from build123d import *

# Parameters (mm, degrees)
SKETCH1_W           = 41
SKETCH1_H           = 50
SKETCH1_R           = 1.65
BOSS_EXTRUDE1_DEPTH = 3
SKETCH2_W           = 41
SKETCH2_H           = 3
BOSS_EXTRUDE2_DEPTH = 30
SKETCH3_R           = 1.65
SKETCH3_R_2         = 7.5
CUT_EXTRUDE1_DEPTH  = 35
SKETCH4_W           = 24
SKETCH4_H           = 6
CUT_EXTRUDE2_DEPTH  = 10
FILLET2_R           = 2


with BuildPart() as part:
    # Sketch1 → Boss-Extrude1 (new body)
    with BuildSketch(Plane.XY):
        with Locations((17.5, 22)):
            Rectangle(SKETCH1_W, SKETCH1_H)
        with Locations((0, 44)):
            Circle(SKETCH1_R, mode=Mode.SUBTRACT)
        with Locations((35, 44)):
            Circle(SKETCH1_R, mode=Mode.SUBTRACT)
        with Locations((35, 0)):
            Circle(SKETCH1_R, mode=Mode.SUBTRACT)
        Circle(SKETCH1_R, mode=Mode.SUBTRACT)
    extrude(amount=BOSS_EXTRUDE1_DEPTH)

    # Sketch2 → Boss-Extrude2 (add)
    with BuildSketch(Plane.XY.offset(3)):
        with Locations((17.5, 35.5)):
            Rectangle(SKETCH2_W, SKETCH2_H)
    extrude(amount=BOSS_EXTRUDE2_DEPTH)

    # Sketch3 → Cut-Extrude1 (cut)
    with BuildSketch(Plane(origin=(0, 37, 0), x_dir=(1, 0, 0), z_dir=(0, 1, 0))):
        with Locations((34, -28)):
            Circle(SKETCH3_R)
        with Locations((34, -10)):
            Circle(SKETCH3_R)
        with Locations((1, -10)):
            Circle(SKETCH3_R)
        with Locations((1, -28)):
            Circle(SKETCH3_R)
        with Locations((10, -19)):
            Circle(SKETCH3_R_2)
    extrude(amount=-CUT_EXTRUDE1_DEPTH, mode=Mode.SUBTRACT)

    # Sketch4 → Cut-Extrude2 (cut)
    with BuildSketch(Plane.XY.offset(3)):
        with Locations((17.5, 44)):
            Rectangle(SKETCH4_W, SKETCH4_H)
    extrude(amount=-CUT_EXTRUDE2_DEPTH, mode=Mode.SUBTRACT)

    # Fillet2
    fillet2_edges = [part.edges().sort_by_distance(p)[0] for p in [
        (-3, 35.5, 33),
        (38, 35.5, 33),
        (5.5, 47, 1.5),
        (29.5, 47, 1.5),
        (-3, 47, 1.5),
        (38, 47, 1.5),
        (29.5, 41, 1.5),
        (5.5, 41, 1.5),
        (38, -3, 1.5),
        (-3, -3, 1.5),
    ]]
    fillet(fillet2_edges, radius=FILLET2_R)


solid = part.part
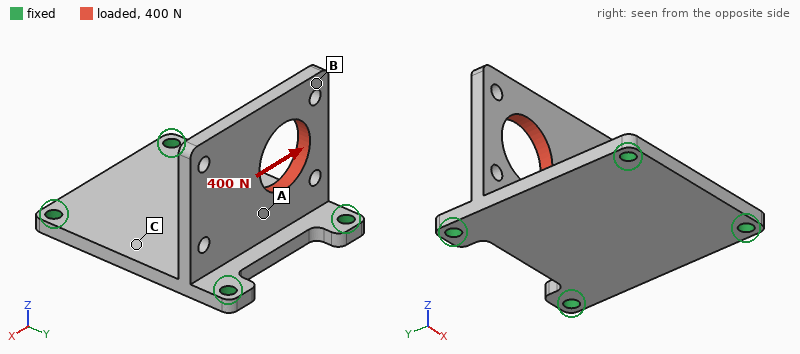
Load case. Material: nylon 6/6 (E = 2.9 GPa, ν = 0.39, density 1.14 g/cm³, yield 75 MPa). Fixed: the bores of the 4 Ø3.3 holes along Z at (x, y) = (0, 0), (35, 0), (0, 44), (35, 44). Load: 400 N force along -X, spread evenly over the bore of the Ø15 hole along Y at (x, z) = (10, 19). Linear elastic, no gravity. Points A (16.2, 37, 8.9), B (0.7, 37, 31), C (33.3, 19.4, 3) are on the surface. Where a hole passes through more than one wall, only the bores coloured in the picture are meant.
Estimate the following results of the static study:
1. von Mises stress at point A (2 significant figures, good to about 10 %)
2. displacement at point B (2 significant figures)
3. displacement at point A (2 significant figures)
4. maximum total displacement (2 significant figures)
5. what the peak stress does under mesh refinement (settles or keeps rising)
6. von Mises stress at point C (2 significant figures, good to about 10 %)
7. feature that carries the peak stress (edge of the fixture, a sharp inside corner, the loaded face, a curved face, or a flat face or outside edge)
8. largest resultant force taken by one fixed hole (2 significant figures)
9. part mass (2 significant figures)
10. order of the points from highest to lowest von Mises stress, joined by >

14 MPa
0.73 mm
0.19 mm
0.81 mm
keeps rising
7.0 MPa
edge of the fixture
250 N
9.9 g
A > C > B
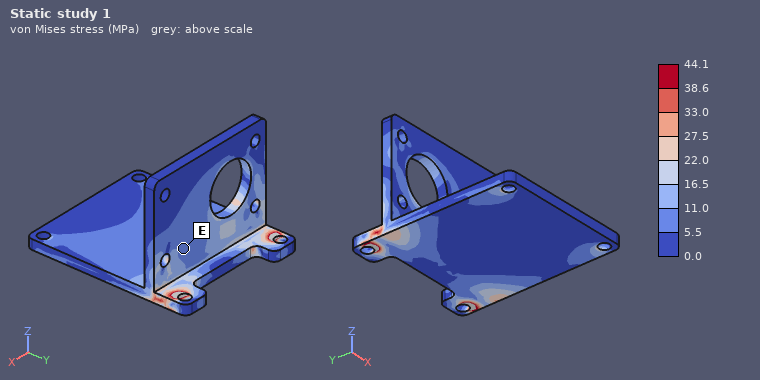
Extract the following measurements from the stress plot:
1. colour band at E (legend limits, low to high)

5.5 to 11.0 MPa
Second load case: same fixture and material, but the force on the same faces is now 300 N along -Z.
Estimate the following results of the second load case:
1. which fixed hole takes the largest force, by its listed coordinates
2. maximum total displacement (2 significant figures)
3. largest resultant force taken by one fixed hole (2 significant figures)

(0, 44)
0.74 mm
190 N
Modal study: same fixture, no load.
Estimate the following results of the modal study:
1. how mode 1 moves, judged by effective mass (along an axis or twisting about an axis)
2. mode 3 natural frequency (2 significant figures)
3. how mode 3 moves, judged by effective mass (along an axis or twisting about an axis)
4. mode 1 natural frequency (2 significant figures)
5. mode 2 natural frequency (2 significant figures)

along Y
2000 Hz
along Z
660 Hz
1300 Hz
